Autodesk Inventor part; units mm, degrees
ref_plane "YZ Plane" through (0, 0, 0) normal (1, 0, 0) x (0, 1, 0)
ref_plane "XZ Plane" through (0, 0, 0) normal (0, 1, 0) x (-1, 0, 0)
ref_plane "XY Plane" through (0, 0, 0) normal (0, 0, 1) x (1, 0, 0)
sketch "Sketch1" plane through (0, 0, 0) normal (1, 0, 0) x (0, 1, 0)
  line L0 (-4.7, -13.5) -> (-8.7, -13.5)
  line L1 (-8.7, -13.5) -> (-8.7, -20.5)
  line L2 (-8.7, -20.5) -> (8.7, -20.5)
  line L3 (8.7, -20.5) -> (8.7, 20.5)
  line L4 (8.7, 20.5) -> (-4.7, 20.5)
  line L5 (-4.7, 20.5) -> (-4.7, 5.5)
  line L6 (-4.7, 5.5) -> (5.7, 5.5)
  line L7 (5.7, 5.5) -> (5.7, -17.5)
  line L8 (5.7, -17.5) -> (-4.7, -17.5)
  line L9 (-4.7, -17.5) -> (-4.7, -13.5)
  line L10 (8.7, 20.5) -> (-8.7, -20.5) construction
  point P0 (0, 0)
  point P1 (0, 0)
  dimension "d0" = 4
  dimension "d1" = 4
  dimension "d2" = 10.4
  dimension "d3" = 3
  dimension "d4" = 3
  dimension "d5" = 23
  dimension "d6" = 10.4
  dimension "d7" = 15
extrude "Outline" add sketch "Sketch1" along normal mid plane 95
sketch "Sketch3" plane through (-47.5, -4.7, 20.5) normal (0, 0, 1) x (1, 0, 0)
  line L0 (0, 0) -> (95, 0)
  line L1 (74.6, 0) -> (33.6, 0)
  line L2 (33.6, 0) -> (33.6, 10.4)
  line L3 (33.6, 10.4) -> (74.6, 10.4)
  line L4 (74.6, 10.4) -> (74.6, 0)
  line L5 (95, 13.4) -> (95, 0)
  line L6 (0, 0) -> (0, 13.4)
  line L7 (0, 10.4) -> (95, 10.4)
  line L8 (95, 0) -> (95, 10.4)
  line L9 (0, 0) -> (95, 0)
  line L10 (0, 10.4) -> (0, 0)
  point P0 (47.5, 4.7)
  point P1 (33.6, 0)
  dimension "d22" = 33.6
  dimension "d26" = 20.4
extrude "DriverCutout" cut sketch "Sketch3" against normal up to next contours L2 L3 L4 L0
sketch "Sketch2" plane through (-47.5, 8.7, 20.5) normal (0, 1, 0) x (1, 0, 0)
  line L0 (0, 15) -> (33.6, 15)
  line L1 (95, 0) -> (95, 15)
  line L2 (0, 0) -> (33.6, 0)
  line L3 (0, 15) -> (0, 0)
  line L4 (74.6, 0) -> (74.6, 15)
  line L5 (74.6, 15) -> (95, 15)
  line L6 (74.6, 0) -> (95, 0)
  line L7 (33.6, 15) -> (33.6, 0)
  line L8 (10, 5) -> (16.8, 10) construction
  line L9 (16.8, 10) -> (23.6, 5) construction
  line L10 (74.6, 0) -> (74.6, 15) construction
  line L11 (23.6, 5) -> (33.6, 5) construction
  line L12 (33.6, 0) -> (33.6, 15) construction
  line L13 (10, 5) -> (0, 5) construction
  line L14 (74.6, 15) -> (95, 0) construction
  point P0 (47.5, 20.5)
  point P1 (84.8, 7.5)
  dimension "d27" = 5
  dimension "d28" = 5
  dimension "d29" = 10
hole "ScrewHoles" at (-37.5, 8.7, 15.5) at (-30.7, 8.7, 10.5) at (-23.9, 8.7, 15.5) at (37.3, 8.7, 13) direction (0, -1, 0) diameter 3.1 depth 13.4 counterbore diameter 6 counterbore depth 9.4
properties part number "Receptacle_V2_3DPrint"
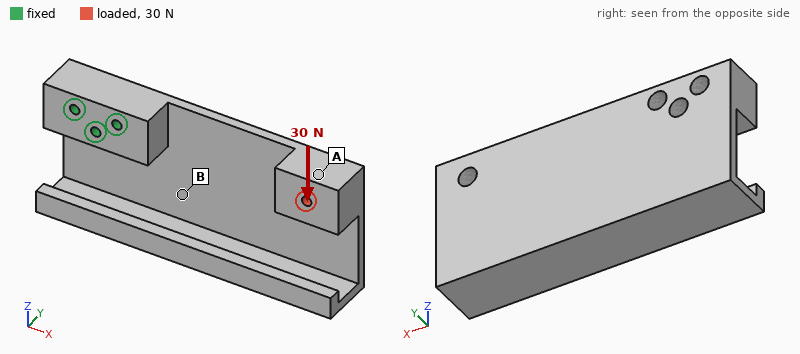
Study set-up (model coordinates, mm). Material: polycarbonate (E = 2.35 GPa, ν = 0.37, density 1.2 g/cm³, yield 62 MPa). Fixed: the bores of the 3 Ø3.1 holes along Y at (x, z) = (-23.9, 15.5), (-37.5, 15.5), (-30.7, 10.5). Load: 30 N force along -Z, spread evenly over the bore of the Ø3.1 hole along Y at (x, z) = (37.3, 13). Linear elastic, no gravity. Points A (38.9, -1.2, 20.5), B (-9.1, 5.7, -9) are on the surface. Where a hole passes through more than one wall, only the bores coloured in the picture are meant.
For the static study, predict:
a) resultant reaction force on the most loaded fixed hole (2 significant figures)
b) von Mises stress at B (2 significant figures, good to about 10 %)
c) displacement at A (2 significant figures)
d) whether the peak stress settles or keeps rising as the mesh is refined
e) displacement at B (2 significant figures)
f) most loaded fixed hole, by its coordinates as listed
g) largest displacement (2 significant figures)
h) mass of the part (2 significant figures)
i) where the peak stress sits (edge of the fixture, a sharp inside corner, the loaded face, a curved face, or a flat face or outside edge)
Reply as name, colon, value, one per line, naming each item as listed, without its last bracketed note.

resultant reaction force on the most loaded fixed hole: 120 N
von Mises stress at B: 1.7 MPa
displacement at A: 0.89 mm
whether the peak stress settles or keeps rising as the mesh is refined: keeps rising
displacement at B: 0.17 mm
most loaded fixed hole, by its coordinates as listed: (-23.9, 15.5)
largest displacement: 1.0 mm
mass of the part: 29 g
where the peak stress sits: edge of the fixture
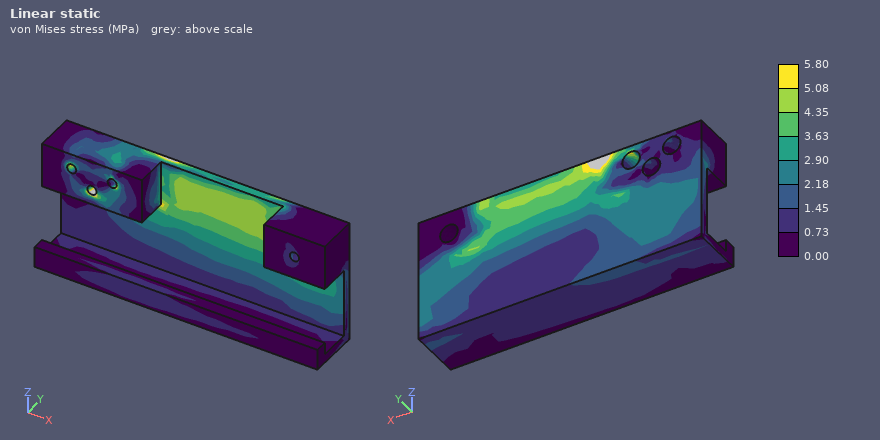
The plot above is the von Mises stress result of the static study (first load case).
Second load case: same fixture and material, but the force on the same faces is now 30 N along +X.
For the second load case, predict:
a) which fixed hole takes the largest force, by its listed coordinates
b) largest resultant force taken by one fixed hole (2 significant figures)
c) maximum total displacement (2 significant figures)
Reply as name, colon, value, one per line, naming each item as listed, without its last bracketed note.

which fixed hole takes the largest force, by its listed coordinates: (-30.7, 10.5)
largest resultant force taken by one fixed hole: 18 N
maximum total displacement: 1.1 mm
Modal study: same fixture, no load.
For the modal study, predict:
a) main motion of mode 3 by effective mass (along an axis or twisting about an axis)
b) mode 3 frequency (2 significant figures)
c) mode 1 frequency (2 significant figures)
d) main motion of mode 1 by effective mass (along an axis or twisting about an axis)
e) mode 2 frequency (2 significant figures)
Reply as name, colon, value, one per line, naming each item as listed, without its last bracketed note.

main motion of mode 3 by effective mass: along Z
mode 3 frequency: 500 Hz
mode 1 frequency: 150 Hz
main motion of mode 1 by effective mass: along Y
mode 2 frequency: 270 Hz
